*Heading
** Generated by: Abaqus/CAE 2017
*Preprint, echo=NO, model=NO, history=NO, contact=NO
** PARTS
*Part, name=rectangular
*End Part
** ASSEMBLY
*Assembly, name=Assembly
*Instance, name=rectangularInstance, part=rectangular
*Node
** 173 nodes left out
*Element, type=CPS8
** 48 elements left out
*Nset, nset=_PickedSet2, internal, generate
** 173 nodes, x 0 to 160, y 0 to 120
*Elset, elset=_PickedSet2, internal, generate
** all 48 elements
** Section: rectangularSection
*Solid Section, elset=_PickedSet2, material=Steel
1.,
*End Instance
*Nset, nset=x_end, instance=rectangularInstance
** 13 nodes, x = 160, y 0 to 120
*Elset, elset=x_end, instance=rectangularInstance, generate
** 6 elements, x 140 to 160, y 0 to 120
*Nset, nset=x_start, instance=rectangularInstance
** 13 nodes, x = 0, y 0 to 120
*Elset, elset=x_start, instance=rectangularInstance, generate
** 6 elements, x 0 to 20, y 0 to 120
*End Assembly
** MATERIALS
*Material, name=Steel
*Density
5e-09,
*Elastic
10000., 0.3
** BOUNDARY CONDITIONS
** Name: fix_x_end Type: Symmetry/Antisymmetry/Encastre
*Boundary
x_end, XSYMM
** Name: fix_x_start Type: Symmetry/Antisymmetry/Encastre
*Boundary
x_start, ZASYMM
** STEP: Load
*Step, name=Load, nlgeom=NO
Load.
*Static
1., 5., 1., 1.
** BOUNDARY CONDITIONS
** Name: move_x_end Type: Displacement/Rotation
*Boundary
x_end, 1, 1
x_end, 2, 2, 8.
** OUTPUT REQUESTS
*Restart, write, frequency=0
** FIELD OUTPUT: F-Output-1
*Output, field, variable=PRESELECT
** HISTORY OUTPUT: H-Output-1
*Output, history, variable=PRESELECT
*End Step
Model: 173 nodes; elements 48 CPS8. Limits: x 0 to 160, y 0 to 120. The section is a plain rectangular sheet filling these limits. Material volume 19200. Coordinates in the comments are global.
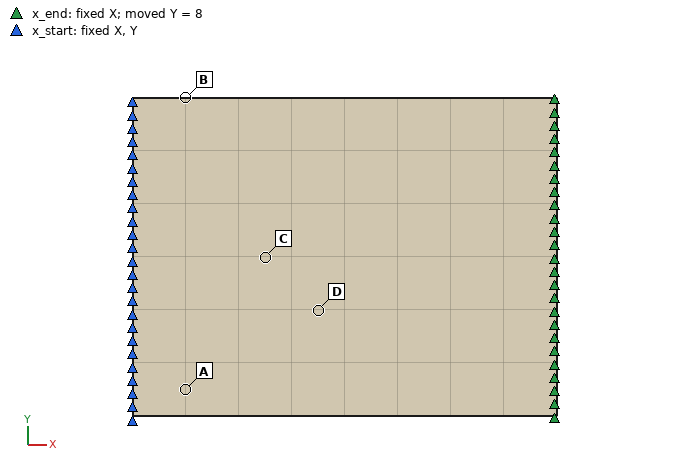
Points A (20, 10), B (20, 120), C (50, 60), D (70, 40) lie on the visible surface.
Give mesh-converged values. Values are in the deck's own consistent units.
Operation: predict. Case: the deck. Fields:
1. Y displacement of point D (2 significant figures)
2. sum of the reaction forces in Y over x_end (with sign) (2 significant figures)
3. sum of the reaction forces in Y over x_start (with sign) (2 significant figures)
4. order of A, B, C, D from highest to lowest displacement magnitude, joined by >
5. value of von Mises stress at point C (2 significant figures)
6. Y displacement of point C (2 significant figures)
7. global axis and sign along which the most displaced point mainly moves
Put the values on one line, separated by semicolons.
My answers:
3.4; 13000; -13000; D > C > B > A; 270; 2.2; +Y
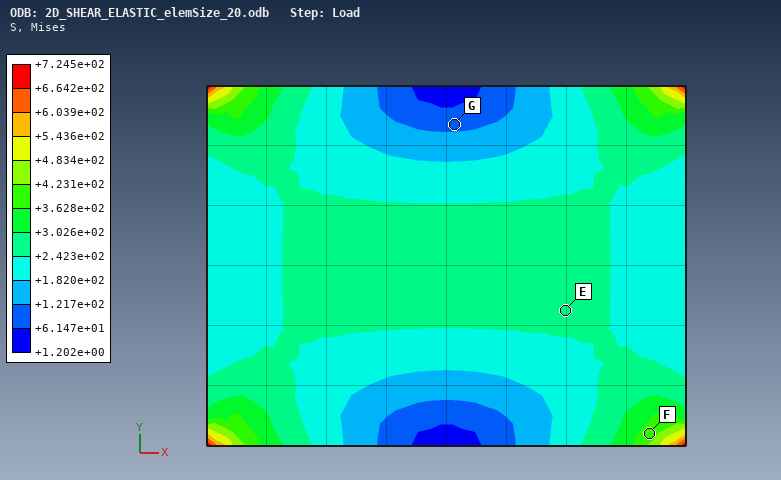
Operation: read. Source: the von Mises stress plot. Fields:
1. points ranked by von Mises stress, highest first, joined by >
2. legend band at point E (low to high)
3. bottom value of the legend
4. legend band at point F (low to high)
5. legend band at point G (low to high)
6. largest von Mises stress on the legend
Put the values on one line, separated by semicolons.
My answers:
F > E > G; +2.423e+02 to +3.026e+02; +1.202e+00; +3.628e+02 to +4.231e+02; +6.147e+01 to +1.217e+02; +7.245e+02
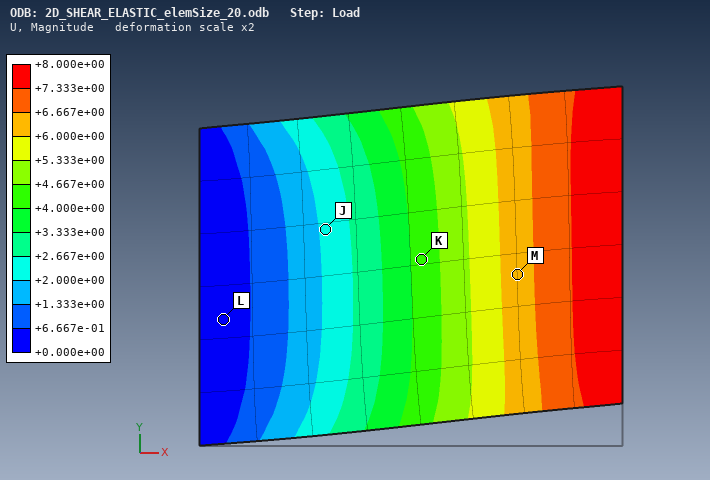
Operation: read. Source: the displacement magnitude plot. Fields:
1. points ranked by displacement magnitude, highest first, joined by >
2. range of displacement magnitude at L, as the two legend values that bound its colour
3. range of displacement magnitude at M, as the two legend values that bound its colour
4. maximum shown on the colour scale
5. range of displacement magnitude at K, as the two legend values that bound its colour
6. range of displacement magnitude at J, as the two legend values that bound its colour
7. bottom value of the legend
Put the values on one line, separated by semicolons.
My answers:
M > K > J > L; +0.000e+00 to +6.667e-01; +6.000e+00 to +6.667e+00; +8.000e+00; +4.000e+00 to +4.667e+00; +2.000e+00 to +2.667e+00; +0.000e+00
